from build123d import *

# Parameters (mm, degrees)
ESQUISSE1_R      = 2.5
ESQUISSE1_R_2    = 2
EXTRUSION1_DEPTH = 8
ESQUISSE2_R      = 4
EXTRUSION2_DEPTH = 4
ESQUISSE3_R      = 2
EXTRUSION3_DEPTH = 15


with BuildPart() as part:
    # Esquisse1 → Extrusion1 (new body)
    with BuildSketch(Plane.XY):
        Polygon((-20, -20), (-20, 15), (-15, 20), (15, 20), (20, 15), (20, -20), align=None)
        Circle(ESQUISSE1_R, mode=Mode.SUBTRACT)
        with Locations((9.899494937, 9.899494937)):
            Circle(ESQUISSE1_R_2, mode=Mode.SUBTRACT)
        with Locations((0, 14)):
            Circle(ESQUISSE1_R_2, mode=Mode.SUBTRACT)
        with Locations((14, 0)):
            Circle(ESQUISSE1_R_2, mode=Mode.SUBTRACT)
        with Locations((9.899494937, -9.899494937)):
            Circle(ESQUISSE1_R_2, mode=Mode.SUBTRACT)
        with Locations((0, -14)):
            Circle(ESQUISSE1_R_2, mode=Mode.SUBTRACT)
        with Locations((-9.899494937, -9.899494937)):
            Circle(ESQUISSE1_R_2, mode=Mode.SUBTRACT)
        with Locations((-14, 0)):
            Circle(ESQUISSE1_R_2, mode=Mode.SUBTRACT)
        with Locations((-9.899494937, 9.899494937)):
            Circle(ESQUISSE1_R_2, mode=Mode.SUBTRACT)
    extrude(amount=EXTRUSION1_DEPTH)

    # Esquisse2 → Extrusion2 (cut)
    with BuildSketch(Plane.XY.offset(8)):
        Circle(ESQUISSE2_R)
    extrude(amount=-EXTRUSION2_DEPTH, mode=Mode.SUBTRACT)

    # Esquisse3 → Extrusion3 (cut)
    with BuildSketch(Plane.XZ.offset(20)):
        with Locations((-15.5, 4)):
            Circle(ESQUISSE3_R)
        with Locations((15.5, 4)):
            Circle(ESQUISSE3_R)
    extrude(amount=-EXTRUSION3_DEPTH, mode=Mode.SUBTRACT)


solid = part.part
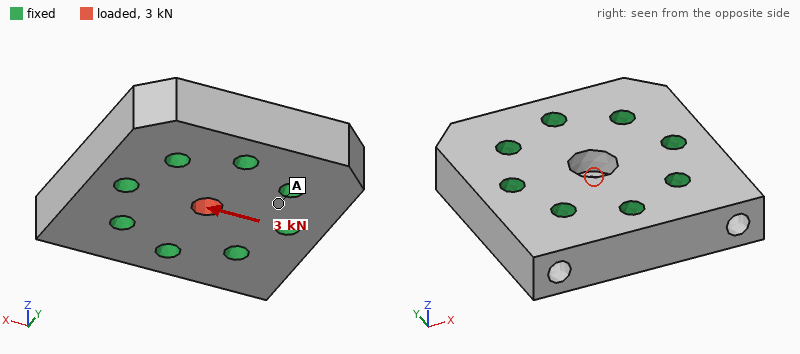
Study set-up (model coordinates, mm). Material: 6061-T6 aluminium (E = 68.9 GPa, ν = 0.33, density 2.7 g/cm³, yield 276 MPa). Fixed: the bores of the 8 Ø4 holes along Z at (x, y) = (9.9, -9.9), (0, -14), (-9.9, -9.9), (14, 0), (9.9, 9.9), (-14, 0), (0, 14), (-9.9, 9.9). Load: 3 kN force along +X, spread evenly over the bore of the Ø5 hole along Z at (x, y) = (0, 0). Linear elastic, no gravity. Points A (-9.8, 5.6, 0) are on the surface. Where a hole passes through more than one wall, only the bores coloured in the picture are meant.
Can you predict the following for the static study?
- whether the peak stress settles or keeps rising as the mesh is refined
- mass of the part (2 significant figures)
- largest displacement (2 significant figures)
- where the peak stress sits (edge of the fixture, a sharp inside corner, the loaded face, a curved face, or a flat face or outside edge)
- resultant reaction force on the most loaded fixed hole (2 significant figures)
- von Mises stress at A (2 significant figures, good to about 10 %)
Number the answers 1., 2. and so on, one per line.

1. keeps rising
2. 30 g
3. 4.4 µm
4. a sharp inside corner
5. 690 N
6. 8.7 MPa
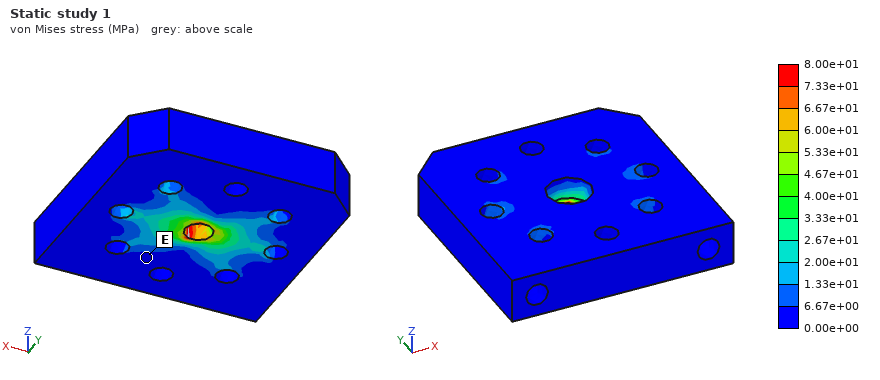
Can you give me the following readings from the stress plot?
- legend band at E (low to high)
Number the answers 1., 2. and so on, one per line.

1. 0.00e+00 to 6.67e+00 MPa
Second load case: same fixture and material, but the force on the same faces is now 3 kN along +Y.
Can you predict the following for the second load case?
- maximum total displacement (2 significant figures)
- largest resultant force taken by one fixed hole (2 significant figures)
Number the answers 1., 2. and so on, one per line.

1. 4.3 µm
2. 690 N
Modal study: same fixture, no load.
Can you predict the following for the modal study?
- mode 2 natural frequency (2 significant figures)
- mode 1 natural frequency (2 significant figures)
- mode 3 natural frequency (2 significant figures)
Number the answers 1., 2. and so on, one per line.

1. 41 kHz
2. 41 kHz
3. 52 kHz
